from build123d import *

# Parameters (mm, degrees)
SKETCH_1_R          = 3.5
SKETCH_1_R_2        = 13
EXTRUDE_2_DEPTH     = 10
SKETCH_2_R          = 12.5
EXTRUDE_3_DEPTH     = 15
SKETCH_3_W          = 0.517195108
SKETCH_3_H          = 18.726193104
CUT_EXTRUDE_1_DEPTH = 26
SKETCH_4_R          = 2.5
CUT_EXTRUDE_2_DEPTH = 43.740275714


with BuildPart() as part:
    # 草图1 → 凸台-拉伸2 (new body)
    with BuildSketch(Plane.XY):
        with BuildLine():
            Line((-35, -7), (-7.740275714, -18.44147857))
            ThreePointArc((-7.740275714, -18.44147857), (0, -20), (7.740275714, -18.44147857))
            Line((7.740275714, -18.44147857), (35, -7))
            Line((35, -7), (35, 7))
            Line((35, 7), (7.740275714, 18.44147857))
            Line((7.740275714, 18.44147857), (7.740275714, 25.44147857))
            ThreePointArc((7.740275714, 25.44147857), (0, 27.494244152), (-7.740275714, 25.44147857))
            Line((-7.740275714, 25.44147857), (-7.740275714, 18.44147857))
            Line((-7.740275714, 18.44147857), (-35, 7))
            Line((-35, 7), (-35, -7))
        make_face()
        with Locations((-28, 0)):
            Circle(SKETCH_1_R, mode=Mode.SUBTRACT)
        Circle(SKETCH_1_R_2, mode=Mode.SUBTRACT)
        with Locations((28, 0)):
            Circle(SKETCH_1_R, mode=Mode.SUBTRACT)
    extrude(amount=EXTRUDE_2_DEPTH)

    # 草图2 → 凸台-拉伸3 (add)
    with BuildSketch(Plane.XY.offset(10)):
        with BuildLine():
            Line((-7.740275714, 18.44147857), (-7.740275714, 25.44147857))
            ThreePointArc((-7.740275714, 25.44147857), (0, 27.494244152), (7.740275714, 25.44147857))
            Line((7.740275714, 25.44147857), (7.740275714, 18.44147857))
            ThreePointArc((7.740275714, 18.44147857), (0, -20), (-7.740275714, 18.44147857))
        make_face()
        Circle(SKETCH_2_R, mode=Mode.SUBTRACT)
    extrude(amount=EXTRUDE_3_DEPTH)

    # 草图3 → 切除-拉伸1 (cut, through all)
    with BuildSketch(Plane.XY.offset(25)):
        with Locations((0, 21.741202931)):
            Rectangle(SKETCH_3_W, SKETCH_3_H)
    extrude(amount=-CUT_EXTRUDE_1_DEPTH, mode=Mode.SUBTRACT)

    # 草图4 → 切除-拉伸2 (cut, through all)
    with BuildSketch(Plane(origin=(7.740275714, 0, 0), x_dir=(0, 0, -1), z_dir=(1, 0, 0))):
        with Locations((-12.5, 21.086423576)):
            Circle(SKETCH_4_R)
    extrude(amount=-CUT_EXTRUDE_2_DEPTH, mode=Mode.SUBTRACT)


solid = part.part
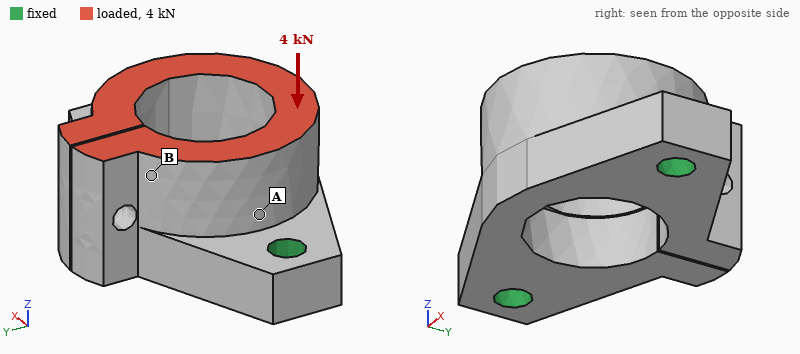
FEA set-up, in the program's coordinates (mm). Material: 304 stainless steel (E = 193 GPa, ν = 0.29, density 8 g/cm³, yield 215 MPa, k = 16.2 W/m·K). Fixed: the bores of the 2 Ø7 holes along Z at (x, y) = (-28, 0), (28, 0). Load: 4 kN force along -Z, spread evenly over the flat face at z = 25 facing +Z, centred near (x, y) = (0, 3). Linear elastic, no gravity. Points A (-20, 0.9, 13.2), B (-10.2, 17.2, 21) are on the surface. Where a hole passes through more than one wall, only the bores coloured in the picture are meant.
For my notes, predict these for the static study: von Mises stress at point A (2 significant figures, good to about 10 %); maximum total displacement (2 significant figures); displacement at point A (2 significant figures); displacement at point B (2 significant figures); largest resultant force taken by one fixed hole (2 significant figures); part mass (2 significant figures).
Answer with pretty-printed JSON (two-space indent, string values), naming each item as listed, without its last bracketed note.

{
  "von Mises stress at point A": "24 MPa",
  "maximum total displacement": "25 µm",
  "displacement at point A": "4.4 µm",
  "displacement at point B": "16 µm",
  "largest resultant force taken by one fixed hole": "2.0 kN",
  "part mass": "220 g"
}
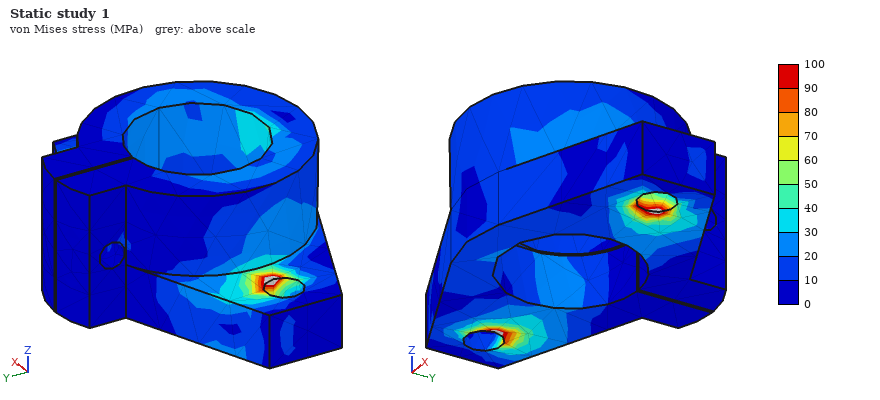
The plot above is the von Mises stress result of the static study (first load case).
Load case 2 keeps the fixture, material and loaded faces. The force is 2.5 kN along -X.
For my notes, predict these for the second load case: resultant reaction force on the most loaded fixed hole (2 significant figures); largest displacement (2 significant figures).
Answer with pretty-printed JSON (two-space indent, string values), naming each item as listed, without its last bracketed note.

{
  "resultant reaction force on the most loaded fixed hole": "1.4 kN",
  "largest displacement": "30 µm"
}
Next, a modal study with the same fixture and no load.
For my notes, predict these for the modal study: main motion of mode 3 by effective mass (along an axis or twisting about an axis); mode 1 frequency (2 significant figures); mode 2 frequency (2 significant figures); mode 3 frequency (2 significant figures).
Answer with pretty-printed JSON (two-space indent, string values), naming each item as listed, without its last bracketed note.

{
  "main motion of mode 3 by effective mass": "along Y",
  "mode 1 frequency": "5600 Hz",
  "mode 2 frequency": "5600 Hz",
  "mode 3 frequency": "6100 Hz"
}
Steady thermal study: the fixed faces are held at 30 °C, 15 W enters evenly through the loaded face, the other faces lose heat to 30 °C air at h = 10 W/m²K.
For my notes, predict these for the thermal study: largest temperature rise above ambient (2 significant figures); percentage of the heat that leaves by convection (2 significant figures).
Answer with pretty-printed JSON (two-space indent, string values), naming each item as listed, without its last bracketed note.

{
  "largest temperature rise above ambient": "47 K",
  "percentage of the heat that leaves by convection": "15 %"
}
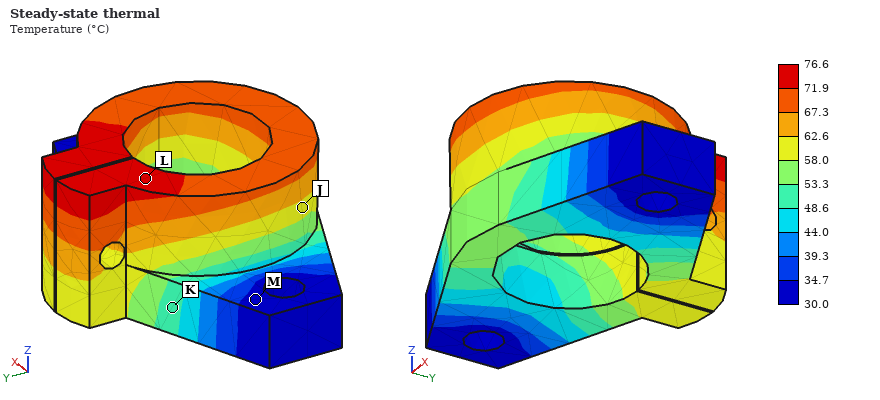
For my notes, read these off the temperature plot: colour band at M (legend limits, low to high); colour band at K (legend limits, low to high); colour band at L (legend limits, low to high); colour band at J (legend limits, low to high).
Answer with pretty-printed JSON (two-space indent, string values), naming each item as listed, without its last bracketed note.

{
  "colour band at M": "30.0 to 34.7 °C",
  "colour band at K": "48.6 to 53.3 °C",
  "colour band at L": "71.9 to 76.6 °C",
  "colour band at J": "58.0 to 62.6 °C"
}
